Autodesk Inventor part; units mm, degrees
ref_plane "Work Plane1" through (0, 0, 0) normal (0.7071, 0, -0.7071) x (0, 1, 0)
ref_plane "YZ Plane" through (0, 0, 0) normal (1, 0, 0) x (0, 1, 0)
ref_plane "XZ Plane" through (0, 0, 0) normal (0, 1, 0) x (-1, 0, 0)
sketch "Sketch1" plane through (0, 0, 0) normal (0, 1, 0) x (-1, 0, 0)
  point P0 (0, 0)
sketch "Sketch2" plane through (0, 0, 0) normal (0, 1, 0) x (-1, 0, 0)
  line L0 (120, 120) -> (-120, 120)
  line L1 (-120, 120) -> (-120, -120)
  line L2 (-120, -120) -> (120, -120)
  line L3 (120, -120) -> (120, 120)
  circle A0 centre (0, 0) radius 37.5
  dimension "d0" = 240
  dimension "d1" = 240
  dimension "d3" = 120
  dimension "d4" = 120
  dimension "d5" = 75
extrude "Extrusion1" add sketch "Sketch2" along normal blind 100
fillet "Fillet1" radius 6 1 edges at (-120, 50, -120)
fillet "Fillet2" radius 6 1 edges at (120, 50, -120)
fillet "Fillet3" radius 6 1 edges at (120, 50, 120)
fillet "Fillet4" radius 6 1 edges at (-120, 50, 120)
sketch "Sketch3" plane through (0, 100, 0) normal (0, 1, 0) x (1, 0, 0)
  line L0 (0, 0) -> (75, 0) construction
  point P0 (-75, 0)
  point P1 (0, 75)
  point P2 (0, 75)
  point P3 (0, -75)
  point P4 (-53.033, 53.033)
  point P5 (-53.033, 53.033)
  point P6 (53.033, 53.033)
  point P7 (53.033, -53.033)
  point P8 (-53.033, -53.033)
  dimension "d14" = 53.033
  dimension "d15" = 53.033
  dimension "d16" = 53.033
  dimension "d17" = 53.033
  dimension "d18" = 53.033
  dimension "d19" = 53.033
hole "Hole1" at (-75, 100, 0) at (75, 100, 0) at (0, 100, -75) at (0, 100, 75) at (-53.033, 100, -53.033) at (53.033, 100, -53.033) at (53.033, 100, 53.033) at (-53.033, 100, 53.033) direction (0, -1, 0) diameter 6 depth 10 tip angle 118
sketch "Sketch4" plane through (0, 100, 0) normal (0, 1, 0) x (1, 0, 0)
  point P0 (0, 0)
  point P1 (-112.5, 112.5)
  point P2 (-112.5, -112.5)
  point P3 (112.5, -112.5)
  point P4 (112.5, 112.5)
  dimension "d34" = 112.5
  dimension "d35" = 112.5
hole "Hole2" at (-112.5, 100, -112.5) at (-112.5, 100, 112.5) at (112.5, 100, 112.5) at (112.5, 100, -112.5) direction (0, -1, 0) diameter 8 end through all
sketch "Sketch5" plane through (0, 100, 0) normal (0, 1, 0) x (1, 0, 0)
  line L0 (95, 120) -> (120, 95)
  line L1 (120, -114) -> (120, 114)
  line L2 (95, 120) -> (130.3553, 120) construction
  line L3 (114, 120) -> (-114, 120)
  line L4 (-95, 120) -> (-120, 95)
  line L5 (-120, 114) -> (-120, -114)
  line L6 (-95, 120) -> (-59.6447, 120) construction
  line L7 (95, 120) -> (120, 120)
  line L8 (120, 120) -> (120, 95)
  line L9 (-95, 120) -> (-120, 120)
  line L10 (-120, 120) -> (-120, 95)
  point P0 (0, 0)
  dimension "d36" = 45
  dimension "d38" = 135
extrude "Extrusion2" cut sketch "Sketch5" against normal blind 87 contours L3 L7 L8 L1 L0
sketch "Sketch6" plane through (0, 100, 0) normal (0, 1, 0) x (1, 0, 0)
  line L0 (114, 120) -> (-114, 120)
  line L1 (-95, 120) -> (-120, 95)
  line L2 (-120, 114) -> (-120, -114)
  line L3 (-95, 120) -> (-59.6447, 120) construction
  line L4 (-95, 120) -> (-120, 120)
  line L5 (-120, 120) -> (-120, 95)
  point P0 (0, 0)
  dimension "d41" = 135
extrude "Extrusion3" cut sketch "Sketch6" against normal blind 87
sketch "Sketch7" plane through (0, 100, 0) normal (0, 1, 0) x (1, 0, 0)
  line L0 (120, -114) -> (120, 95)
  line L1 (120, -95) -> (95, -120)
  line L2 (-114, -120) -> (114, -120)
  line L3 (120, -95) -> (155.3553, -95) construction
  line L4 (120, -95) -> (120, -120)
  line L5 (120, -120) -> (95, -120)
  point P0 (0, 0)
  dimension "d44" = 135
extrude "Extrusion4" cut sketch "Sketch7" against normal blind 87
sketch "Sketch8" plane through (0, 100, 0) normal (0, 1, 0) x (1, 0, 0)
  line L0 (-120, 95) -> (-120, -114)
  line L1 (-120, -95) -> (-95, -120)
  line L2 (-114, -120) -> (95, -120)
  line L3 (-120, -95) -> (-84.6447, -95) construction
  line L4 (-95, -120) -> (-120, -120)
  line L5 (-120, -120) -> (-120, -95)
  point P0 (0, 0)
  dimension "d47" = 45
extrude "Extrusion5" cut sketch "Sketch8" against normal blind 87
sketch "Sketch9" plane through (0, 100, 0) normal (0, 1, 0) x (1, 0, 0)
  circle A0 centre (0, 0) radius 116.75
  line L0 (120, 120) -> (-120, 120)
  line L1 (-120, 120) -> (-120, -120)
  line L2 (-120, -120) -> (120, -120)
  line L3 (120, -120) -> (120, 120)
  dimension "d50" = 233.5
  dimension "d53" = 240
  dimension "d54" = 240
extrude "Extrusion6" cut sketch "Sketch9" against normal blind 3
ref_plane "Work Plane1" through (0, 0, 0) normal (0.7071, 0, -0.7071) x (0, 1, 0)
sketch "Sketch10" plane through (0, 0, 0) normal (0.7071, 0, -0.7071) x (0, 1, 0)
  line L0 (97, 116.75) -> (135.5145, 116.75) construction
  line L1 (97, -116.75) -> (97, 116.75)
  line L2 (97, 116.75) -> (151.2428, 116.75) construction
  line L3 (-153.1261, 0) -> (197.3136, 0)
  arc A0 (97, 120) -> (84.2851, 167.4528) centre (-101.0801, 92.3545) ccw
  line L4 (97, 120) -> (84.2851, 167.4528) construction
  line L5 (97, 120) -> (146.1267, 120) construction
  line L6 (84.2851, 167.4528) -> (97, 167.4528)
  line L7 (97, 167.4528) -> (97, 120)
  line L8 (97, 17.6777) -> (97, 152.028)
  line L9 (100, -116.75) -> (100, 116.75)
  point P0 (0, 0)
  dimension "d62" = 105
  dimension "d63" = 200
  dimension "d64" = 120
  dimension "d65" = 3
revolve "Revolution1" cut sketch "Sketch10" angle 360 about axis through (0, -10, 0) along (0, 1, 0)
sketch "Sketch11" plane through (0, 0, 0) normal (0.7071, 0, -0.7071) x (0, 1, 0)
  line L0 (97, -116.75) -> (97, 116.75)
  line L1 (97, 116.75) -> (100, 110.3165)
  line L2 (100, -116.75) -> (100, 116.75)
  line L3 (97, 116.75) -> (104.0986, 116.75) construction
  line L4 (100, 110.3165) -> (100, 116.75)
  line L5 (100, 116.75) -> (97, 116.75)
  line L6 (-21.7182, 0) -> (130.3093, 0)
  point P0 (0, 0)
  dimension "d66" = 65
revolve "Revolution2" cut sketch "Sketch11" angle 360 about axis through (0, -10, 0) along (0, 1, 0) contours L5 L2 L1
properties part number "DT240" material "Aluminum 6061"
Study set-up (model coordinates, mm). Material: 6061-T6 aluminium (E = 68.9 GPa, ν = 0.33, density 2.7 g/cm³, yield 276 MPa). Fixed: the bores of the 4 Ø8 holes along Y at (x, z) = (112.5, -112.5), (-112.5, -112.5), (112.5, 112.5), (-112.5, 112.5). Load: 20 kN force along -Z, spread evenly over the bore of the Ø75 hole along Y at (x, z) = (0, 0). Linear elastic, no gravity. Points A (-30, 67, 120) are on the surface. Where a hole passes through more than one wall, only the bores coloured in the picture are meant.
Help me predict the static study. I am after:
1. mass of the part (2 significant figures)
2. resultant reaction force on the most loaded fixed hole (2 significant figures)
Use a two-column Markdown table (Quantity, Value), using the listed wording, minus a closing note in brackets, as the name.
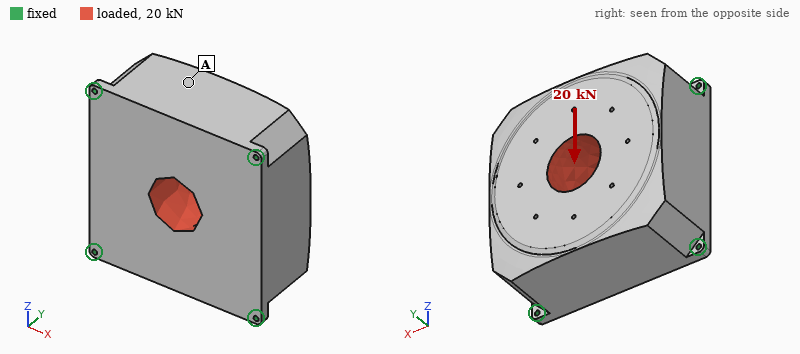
| Quantity | Value |
|---|---|
| mass of the part | 14 kg |
| resultant reaction force on the most loaded fixed hole | 5.8 kN |
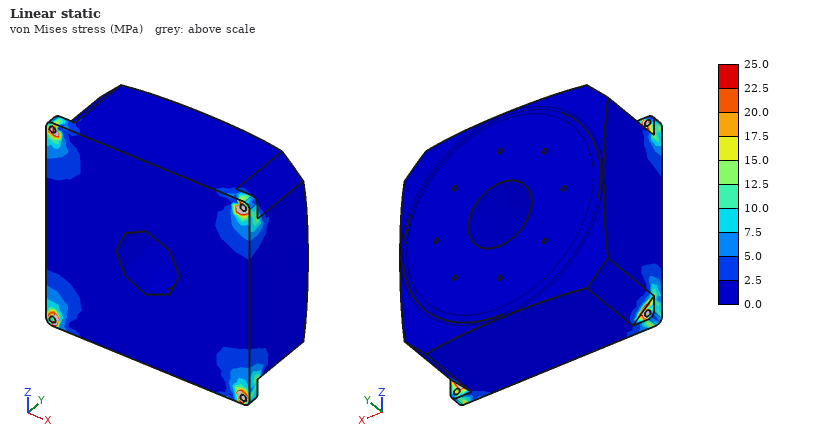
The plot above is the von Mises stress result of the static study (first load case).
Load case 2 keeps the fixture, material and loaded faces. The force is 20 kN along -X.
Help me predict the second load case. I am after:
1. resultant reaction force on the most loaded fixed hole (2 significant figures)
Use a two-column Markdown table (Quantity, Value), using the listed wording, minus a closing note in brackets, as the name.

| Quantity | Value |
|---|---|
| resultant reaction force on the most loaded fixed hole | 5.7 kN |
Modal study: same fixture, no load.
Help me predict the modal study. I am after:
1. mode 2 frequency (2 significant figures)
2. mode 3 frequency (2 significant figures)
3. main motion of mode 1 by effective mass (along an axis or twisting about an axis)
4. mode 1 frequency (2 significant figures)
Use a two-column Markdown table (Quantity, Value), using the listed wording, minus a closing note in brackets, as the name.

| Quantity | Value |
|---|---|
| mode 2 frequency | 2000 Hz |
| mode 3 frequency | 2000 Hz |
| main motion of mode 1 by effective mass | along Y |
| mode 1 frequency | 1700 Hz |
